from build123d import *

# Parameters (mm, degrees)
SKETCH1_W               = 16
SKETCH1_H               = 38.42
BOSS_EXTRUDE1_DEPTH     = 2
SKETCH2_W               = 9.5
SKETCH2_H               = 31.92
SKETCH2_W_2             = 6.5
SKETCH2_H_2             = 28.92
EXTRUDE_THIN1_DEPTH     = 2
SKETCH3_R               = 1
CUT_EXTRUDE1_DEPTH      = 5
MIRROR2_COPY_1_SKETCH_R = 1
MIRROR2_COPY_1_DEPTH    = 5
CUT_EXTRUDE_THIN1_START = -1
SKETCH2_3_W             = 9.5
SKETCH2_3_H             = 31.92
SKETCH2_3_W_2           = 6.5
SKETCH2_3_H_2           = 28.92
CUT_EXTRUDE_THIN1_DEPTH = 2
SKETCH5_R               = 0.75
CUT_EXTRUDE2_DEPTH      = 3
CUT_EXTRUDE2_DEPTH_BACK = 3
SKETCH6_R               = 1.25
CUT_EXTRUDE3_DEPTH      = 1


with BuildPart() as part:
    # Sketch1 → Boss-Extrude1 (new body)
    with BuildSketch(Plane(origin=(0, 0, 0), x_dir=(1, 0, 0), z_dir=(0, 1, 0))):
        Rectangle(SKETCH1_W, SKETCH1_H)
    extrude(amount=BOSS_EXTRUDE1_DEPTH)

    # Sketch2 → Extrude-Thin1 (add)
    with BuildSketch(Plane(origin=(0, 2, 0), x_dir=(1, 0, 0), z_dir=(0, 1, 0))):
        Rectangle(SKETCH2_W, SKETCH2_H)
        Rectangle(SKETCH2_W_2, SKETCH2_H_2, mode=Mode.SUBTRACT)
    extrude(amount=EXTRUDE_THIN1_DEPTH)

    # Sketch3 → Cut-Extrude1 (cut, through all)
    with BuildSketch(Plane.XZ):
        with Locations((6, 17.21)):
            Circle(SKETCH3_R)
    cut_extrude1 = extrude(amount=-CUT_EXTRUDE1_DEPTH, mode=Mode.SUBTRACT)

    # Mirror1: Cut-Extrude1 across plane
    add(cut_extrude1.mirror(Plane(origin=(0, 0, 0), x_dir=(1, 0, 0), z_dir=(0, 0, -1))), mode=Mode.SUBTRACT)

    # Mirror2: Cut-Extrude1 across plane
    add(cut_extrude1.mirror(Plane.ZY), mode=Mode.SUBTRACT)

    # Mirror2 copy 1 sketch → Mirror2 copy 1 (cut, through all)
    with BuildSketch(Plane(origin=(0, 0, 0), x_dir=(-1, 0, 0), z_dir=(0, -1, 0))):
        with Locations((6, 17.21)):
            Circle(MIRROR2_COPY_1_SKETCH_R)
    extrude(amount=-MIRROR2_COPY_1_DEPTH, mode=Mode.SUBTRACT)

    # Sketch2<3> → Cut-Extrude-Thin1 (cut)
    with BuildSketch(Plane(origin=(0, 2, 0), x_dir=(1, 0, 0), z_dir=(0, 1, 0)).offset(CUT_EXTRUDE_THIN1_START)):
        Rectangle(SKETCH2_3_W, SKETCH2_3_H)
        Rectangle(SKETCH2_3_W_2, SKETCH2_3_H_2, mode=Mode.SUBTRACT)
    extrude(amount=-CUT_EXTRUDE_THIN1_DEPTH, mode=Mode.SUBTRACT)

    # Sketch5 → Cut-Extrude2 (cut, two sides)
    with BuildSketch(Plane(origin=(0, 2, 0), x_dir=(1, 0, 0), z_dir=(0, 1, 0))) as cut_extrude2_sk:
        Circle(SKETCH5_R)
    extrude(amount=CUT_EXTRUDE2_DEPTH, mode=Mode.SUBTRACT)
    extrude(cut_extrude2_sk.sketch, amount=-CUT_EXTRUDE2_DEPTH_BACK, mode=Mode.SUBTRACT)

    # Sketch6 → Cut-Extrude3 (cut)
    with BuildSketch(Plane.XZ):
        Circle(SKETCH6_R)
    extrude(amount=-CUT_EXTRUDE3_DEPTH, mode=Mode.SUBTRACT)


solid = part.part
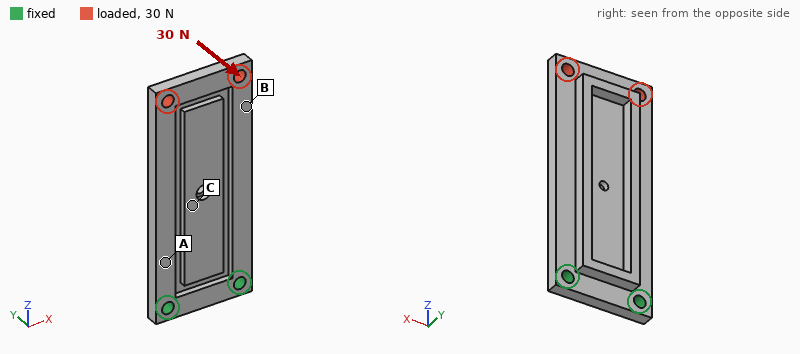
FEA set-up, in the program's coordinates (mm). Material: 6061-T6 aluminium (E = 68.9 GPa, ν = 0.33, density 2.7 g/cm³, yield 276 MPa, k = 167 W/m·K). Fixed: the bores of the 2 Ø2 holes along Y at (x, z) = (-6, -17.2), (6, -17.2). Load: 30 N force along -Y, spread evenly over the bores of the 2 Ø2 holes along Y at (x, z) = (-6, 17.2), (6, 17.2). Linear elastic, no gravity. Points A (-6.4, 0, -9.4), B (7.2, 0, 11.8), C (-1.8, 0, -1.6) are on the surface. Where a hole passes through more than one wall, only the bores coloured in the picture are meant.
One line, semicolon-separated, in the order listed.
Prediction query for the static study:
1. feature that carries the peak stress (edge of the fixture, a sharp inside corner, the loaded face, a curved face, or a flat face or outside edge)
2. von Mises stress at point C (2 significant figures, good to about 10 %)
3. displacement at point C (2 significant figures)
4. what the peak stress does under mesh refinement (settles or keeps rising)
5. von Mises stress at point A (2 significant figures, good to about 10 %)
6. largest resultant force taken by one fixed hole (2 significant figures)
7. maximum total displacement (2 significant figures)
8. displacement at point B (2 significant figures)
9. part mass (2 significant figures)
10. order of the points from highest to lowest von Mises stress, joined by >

edge of the fixture; 31 MPa; 0.11 mm; keeps rising; 45 MPa; 17 N; 0.37 mm; 0.27 mm; 3.5 g; A > C > B
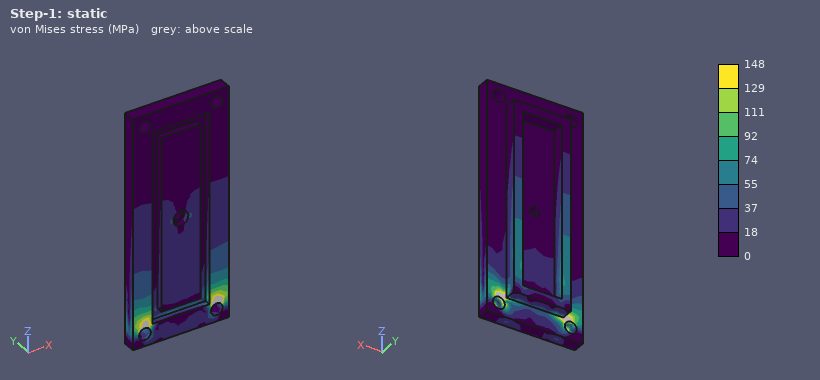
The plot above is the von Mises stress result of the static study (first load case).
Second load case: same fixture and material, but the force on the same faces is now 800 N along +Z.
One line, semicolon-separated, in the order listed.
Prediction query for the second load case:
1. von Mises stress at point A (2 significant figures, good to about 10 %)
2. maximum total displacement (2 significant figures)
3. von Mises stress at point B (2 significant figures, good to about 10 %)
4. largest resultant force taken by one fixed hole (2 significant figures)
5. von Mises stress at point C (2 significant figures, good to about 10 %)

45 MPa; 0.12 mm; 54 MPa; 400 N; 45 MPa
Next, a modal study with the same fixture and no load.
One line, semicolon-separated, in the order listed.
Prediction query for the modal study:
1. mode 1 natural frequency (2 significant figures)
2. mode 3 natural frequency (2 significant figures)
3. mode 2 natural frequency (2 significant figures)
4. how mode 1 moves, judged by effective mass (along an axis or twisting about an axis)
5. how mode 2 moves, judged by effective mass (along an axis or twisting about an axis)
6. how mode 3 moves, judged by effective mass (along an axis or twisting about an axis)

1500 Hz; 8300 Hz; 5400 Hz; along Y; twisting about Z; along X
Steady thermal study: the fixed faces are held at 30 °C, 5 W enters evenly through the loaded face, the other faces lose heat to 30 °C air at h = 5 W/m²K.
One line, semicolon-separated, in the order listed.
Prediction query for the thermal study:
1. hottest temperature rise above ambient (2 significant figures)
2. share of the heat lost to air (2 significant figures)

34 K; 3.0 %
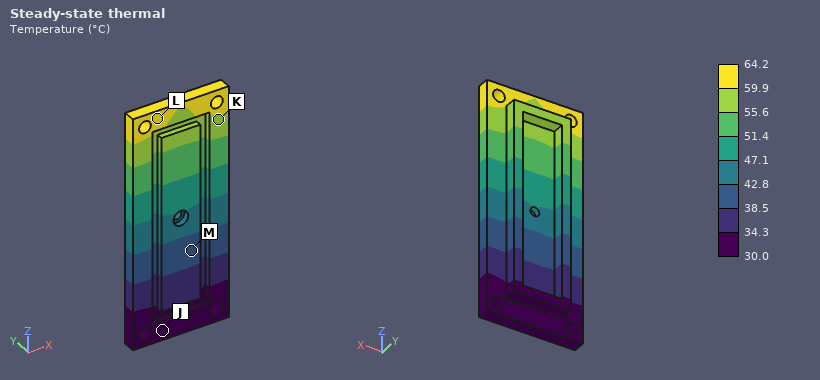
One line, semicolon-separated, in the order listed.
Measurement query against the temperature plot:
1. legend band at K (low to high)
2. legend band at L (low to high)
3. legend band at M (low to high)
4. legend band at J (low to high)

55.6 to 59.9 °C; 59.9 to 64.2 °C; 38.5 to 42.8 °C; 30.0 to 34.3 °C
